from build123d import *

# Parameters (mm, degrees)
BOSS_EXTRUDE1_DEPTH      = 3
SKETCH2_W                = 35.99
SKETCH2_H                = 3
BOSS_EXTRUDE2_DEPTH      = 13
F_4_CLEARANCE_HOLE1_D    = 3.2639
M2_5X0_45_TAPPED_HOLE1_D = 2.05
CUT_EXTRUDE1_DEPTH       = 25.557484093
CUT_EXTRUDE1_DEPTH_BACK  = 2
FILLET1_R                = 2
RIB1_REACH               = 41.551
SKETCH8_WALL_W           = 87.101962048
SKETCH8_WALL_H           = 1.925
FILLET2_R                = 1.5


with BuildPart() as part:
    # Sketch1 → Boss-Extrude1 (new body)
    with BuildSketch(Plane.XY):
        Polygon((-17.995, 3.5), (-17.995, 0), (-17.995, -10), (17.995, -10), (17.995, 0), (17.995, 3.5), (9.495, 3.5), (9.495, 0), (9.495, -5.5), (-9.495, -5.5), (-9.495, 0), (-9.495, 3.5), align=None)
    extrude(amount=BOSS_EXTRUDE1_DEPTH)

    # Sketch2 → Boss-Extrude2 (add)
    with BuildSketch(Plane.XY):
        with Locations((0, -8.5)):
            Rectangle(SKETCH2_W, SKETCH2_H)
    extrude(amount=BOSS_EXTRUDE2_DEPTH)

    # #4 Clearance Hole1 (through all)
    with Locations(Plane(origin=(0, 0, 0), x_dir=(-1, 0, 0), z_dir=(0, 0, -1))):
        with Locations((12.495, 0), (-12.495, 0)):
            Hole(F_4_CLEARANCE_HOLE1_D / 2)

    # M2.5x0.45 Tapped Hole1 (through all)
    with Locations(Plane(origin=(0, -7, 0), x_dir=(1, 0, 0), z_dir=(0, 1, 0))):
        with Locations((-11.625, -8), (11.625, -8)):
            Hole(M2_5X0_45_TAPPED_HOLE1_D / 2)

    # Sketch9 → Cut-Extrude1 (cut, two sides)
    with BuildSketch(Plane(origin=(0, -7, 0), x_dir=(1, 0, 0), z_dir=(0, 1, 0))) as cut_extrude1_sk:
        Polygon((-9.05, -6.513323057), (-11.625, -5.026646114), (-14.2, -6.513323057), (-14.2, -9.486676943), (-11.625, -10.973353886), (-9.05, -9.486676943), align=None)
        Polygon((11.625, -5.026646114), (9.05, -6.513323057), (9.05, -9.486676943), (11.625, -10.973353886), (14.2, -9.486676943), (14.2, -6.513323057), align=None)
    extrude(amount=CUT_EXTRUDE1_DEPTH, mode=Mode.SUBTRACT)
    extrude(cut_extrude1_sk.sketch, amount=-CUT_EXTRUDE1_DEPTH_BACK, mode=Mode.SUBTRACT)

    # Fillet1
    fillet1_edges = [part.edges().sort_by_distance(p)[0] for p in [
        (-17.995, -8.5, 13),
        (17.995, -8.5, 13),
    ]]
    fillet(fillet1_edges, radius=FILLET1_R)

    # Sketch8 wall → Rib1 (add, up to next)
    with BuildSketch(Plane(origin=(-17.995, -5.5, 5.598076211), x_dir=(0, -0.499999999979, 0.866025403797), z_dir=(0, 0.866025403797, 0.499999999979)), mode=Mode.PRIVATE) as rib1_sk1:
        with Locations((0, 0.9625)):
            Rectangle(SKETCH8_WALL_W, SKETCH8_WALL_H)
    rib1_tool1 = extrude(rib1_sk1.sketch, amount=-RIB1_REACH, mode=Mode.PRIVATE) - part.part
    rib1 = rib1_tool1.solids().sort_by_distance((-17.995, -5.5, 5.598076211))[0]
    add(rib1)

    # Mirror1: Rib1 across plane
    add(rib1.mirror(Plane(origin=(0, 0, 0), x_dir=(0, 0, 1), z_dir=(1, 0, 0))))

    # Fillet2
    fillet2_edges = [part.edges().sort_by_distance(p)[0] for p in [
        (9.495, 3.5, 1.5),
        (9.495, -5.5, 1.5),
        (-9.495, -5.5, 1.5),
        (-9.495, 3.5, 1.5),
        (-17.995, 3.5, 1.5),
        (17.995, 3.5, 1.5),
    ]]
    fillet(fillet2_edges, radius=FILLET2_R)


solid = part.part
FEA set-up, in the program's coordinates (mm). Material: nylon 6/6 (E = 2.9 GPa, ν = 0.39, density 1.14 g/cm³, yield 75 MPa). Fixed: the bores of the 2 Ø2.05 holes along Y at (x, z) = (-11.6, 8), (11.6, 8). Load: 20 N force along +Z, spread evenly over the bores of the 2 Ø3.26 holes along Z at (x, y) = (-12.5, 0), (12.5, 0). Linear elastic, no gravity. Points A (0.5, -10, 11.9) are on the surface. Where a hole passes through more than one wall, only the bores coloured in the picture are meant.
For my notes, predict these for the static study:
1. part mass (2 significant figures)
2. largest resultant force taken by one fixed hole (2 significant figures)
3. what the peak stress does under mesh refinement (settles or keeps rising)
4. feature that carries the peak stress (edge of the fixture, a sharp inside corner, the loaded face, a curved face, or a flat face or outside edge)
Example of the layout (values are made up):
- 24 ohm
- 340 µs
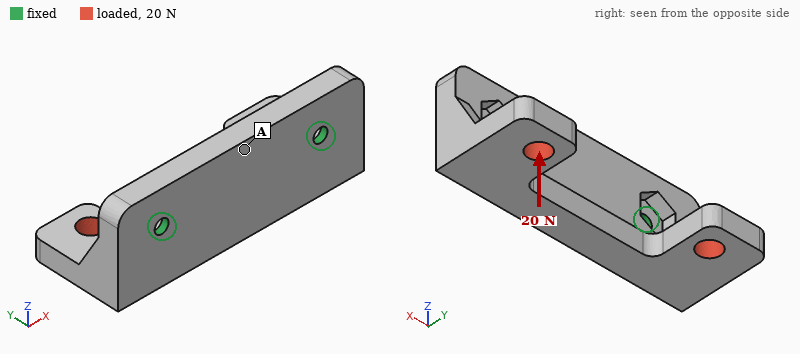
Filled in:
- 2.2 g
- 10 N
- keeps rising
- edge of the fixture
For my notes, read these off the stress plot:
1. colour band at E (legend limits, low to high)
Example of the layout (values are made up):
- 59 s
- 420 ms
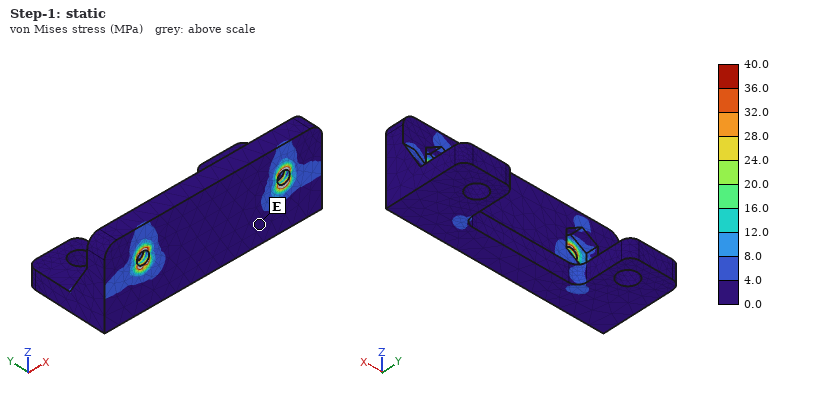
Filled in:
- 0.0 to 4.0 MPa
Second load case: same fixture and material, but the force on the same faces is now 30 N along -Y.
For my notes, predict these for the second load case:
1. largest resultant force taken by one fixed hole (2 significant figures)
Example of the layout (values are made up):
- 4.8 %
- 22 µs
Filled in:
- 15 N
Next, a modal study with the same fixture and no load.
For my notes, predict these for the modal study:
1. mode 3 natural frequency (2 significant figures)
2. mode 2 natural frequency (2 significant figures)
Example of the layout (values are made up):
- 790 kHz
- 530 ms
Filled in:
- 3800 Hz
- 2600 Hz
